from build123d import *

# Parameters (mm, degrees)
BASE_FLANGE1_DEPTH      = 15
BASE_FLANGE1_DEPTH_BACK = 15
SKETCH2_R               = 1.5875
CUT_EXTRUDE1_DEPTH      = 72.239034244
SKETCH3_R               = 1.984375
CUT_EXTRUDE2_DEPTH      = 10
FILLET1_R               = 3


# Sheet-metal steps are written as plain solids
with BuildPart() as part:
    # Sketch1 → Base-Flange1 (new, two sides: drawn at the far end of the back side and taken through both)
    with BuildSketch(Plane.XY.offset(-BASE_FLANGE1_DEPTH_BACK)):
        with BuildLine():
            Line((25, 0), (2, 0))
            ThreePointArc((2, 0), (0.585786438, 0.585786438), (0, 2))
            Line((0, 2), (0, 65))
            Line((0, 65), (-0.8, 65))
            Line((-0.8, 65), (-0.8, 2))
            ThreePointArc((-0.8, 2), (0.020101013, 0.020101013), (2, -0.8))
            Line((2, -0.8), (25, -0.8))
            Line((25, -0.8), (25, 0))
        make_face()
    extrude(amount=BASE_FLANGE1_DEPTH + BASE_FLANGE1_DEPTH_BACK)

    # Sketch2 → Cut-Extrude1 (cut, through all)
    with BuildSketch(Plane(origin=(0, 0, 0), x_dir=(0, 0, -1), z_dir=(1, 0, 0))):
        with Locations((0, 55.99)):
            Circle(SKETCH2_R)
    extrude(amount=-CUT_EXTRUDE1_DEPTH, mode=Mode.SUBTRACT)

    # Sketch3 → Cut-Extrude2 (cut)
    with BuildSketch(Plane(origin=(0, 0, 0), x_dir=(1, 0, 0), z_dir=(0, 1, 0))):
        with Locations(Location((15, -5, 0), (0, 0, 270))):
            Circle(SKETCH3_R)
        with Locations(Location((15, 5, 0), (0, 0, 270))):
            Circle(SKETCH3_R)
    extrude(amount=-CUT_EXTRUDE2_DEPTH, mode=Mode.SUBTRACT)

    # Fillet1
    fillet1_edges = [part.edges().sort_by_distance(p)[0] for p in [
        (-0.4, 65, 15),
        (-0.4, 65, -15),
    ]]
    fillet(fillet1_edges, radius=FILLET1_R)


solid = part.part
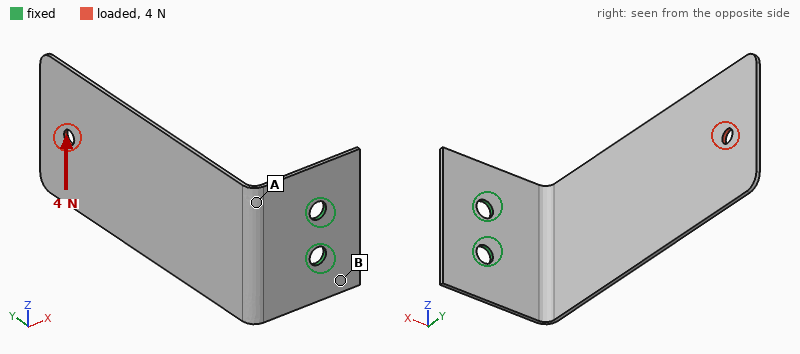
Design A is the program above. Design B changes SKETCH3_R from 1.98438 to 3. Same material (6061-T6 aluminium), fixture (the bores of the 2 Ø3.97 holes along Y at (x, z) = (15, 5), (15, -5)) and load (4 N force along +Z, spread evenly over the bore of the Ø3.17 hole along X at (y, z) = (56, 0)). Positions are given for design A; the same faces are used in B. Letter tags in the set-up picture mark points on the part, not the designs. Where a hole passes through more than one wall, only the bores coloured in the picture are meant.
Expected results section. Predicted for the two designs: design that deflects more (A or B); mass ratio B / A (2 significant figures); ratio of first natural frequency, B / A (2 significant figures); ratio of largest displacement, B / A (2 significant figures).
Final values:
A
0.99
1.0
0.84
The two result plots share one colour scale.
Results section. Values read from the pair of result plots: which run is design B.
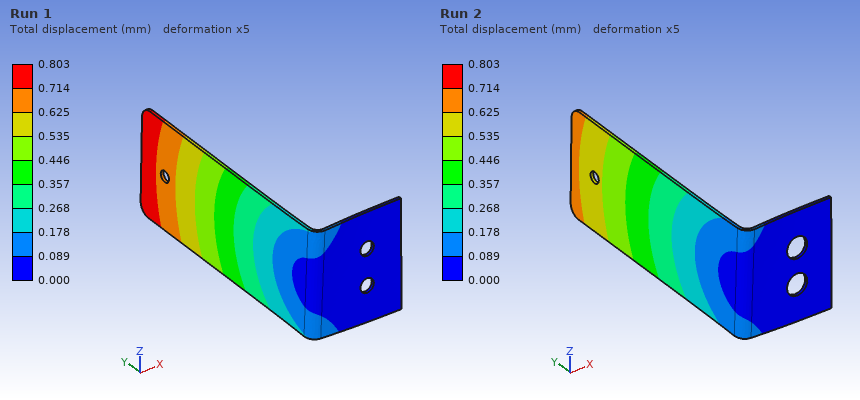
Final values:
Run 2
